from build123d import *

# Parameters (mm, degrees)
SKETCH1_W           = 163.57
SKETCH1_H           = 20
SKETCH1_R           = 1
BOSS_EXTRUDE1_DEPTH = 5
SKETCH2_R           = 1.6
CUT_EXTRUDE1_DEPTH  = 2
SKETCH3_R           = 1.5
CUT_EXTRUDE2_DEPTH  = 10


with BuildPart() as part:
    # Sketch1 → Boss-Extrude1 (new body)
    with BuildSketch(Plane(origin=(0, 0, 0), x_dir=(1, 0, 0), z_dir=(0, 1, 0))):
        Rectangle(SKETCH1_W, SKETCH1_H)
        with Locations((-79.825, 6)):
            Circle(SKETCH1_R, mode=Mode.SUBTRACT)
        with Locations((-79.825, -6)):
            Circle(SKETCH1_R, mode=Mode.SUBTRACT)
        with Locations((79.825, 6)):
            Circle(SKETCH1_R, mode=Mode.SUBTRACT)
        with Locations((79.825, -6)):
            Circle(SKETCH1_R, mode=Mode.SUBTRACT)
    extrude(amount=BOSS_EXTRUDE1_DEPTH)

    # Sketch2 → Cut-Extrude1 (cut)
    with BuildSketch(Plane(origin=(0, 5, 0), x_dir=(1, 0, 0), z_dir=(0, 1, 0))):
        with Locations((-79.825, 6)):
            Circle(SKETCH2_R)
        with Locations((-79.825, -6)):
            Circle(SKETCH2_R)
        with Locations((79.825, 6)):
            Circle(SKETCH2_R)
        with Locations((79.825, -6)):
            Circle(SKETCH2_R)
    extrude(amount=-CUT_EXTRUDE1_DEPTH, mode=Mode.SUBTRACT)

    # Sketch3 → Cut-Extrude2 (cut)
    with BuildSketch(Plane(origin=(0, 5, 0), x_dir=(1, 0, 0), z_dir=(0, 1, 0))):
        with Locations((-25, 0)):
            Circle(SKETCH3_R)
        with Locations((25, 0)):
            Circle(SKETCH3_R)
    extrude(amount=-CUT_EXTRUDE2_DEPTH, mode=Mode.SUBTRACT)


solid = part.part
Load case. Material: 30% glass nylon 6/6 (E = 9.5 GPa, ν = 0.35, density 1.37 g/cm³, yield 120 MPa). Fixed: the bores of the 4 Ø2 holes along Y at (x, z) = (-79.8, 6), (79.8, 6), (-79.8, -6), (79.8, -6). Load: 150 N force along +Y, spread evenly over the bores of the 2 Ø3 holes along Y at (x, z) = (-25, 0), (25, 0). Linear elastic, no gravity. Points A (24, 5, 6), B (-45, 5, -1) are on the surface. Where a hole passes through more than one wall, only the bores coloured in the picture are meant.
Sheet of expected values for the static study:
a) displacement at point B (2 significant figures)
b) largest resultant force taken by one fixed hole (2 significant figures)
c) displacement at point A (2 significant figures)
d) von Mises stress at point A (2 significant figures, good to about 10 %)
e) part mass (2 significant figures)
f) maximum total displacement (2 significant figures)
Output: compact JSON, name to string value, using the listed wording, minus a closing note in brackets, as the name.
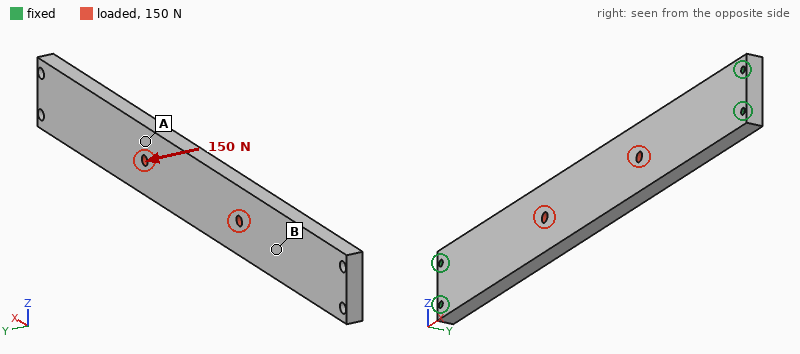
{"displacement at point B": "0.81 mm", "largest resultant force taken by one fixed hole": "71 N", "displacement at point A": "1.3 mm", "von Mises stress at point A": "21 MPa", "part mass": "22 g", "maximum total displacement": "1.6 mm"}
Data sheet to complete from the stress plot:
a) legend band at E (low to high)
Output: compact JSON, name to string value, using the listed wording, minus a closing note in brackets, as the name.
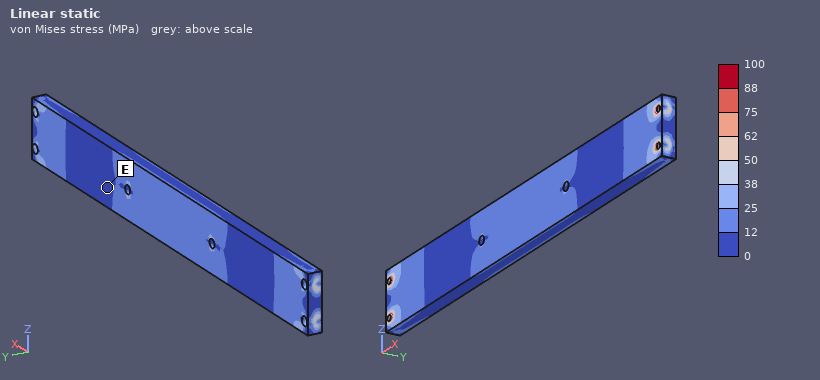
{"legend band at E": "0 to 12 MPa"}
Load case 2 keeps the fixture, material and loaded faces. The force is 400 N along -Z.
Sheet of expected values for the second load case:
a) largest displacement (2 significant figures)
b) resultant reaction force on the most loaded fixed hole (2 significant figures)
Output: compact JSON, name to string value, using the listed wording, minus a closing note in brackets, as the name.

{"largest displacement": "0.30 mm", "resultant reaction force on the most loaded fixed hole": "520 N"}
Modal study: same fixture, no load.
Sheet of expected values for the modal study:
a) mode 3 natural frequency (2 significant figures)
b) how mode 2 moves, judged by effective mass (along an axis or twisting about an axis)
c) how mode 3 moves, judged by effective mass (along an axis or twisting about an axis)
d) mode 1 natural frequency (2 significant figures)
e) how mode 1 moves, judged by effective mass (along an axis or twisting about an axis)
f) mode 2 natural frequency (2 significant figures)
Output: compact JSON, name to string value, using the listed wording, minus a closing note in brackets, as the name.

{"mode 3 natural frequency": "1700 Hz", "how mode 2 moves, judged by effective mass": "twisting about Z", "how mode 3 moves, judged by effective mass": "along Z", "mode 1 natural frequency": "460 Hz", "how mode 1 moves, judged by effective mass": "along Y", "mode 2 natural frequency": "1300 Hz"}
